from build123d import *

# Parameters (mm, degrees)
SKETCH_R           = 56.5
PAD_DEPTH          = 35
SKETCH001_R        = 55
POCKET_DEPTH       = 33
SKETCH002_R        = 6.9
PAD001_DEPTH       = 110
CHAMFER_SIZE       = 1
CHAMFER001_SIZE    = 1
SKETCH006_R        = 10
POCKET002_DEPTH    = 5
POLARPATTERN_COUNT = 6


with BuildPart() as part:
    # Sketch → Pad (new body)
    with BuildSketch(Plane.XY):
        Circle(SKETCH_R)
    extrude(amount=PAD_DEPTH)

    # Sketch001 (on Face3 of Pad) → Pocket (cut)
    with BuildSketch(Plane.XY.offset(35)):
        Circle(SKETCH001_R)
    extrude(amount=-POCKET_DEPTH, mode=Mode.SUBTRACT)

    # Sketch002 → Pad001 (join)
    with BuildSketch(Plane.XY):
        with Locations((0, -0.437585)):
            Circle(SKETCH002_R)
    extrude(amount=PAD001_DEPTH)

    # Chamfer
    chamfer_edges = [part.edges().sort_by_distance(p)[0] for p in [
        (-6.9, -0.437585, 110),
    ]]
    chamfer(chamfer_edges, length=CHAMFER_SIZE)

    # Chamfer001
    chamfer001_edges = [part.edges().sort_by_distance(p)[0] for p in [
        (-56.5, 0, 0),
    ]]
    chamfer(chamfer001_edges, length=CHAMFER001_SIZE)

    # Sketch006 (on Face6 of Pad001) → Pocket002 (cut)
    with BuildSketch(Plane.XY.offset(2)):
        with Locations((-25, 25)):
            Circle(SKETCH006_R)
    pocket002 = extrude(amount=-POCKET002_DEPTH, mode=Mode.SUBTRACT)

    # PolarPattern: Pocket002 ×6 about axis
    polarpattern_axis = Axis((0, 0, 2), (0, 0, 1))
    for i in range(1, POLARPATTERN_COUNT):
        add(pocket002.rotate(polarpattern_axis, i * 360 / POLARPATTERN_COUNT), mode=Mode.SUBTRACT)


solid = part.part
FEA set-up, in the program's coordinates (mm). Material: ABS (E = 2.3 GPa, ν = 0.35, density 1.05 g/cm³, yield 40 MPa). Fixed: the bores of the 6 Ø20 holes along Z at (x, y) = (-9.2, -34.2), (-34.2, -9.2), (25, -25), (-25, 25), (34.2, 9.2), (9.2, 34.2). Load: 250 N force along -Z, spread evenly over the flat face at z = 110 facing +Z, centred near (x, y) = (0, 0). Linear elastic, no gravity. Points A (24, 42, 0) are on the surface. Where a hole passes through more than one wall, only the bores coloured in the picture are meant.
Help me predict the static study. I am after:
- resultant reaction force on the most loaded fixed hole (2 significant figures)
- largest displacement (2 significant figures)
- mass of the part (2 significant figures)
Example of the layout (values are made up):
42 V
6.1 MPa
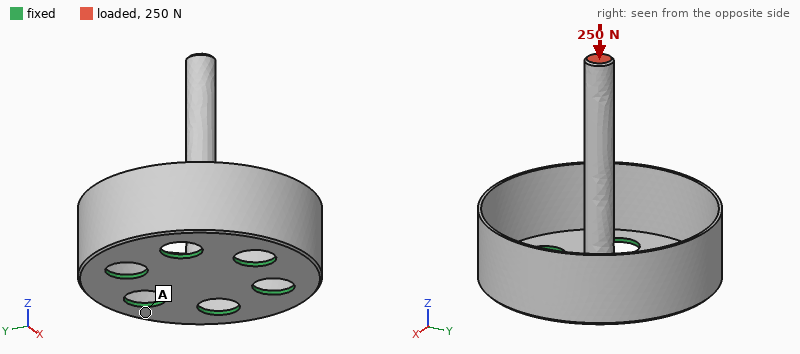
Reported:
49 N
1.1 mm
52 g
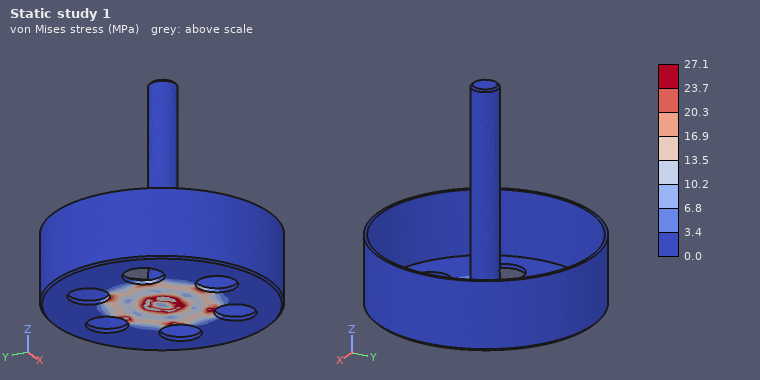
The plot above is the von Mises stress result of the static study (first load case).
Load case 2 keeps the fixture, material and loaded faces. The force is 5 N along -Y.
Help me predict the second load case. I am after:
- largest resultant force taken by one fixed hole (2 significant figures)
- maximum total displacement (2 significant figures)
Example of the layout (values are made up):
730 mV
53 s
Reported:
9.4 N
2.1 mm
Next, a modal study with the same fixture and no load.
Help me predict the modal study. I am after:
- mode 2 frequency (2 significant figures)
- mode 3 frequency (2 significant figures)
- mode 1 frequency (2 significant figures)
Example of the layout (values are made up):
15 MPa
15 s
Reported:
110 Hz
470 Hz
110 Hz
